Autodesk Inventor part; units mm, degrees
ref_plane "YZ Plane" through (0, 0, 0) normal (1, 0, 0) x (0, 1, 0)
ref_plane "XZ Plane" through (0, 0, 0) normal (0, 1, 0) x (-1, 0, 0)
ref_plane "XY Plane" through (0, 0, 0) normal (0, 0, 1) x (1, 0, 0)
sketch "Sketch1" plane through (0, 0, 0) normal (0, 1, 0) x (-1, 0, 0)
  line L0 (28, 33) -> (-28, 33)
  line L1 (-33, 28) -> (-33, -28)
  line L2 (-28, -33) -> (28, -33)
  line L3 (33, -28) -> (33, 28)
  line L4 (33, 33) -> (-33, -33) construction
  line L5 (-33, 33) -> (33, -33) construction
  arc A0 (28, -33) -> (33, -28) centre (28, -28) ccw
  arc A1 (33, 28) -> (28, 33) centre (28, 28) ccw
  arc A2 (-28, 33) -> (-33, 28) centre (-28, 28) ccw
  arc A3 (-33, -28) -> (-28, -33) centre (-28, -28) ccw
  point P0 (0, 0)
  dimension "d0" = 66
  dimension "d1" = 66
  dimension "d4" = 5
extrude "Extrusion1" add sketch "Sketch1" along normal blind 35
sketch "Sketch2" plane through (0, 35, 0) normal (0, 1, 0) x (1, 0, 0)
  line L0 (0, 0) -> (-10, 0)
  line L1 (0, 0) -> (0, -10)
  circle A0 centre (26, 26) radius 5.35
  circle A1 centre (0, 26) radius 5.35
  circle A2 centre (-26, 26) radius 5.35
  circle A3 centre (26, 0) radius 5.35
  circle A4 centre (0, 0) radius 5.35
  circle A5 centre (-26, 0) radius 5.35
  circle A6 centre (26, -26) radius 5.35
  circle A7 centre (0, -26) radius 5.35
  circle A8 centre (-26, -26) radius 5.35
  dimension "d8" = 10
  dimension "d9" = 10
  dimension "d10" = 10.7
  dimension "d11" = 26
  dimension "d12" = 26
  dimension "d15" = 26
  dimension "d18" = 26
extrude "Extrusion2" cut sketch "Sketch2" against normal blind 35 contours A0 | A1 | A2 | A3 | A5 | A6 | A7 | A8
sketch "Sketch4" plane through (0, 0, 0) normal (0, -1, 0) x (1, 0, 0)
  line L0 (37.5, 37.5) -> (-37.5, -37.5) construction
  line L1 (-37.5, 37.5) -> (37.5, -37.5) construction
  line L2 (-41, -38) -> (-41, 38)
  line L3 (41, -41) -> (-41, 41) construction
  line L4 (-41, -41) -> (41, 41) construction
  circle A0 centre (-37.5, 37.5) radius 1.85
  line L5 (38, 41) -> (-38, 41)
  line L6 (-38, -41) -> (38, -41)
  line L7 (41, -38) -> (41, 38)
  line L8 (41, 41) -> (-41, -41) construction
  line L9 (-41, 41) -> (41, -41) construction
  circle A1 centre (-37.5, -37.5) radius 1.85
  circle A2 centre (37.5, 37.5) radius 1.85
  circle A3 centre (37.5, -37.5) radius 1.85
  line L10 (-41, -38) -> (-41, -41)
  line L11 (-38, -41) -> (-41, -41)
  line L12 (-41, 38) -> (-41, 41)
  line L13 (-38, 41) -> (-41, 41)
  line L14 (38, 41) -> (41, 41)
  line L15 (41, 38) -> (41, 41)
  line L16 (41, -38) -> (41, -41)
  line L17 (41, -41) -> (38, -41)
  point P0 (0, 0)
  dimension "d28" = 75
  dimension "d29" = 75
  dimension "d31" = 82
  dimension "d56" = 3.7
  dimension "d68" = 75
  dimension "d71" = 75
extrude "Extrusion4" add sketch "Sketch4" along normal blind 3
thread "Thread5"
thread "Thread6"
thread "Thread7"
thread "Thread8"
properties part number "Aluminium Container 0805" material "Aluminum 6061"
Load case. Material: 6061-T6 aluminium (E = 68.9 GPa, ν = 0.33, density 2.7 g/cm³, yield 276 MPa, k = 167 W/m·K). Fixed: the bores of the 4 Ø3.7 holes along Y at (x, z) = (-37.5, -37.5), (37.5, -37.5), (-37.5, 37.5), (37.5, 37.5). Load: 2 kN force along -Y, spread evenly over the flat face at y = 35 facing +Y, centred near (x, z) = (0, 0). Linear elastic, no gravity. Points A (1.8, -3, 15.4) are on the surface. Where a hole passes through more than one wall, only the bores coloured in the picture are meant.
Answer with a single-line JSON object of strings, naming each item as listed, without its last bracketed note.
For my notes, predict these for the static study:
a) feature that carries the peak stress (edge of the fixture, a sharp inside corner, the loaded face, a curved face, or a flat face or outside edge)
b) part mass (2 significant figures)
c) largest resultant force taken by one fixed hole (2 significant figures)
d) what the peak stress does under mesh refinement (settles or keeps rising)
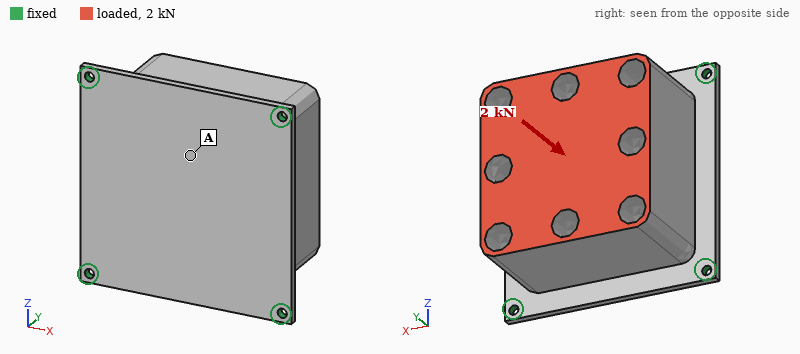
{"feature that carries the peak stress": "edge of the fixture", "part mass": "400 g", "largest resultant force taken by one fixed hole": "550 N", "what the peak stress does under mesh refinement": "keeps rising"}
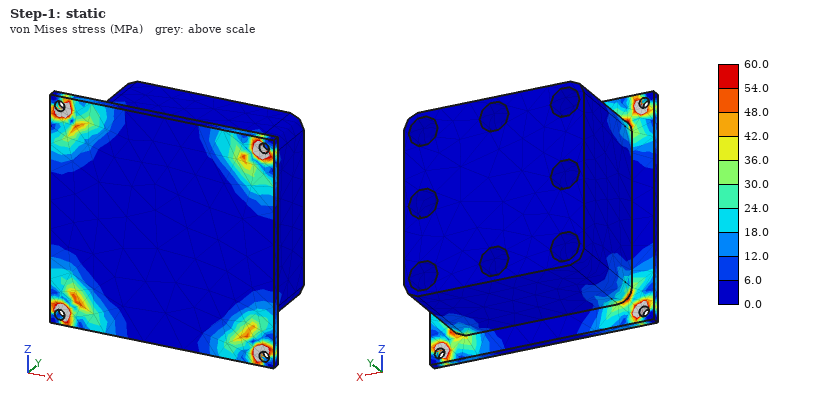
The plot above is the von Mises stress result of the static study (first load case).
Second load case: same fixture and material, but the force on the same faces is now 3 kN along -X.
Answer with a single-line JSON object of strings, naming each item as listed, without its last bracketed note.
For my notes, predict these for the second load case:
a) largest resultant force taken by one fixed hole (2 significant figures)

{"largest resultant force taken by one fixed hole": "1.2 kN"}
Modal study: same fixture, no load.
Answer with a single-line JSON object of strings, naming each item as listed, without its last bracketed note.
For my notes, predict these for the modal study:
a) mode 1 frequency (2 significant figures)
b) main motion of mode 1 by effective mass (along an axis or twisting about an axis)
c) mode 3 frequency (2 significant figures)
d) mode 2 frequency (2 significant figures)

{"mode 1 frequency": "2100 Hz", "main motion of mode 1 by effective mass": "along Y", "mode 3 frequency": "2500 Hz", "mode 2 frequency": "2500 Hz"}
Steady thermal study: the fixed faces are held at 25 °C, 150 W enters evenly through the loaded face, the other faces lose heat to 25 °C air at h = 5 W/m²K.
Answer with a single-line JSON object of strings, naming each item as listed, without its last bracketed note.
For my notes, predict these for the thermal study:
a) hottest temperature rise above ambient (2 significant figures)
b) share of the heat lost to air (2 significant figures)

{"hottest temperature rise above ambient": "72 K", "share of the heat lost to air": "5.9 %"}
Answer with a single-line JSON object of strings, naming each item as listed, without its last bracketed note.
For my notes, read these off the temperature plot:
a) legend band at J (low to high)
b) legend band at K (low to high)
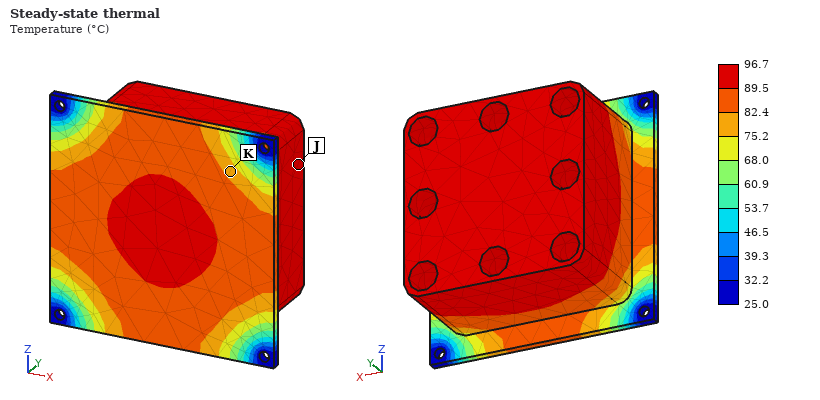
{"legend band at J": "89.5 to 96.7 °C", "legend band at K": "75.2 to 82.4 °C"}
